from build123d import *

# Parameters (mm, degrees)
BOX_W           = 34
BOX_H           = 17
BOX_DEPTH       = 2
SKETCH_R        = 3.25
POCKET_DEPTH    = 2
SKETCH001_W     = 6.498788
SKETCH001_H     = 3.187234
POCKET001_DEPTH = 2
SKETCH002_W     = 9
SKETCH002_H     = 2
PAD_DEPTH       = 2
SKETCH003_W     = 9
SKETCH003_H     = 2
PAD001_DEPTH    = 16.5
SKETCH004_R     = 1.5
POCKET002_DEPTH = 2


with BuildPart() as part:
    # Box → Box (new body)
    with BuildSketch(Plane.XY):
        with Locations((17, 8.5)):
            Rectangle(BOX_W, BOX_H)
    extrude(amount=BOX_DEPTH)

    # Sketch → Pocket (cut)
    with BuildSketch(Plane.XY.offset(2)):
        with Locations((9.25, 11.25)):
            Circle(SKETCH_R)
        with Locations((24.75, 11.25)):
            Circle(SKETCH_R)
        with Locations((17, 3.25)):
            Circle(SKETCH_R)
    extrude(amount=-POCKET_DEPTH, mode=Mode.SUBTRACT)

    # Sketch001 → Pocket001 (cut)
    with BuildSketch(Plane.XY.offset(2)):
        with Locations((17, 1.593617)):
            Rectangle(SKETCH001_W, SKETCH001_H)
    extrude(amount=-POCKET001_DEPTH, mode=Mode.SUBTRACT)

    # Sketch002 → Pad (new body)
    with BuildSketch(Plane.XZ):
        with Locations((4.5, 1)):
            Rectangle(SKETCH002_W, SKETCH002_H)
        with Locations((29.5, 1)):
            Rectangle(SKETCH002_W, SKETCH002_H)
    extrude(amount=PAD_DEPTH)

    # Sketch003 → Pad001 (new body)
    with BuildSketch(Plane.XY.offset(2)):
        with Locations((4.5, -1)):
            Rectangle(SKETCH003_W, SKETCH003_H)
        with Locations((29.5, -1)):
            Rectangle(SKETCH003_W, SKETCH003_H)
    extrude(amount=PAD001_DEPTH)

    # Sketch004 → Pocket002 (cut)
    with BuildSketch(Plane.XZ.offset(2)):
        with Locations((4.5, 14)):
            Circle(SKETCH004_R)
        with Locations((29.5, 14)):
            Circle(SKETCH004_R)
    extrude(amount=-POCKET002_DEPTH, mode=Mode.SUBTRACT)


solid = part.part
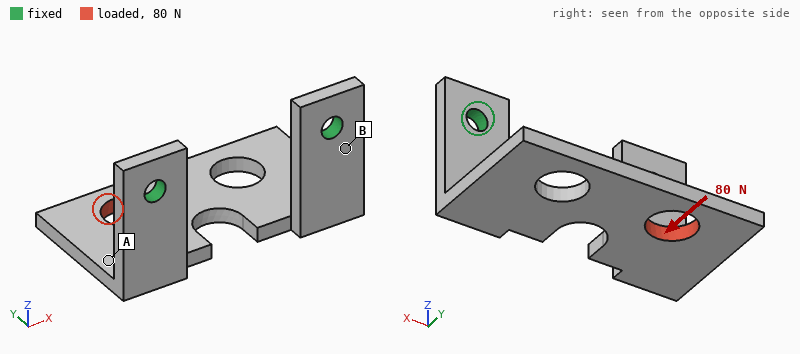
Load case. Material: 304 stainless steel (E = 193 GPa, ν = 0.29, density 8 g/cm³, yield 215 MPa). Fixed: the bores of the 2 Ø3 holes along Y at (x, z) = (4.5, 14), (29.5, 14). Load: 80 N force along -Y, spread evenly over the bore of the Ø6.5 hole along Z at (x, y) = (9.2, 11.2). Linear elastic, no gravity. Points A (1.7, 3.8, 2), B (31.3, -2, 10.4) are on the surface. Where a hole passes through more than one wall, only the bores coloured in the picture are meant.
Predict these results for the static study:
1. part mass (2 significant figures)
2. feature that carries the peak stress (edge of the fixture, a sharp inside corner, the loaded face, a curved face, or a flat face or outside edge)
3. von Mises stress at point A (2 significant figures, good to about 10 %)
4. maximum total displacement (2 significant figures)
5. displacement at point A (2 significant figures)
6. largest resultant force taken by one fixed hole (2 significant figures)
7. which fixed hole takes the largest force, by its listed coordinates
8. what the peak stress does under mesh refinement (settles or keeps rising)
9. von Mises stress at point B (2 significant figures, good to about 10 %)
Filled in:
13 g
edge of the fixture
13 MPa
62 µm
29 µm
60 N
(4.5, 14)
keeps rising
43 MPa
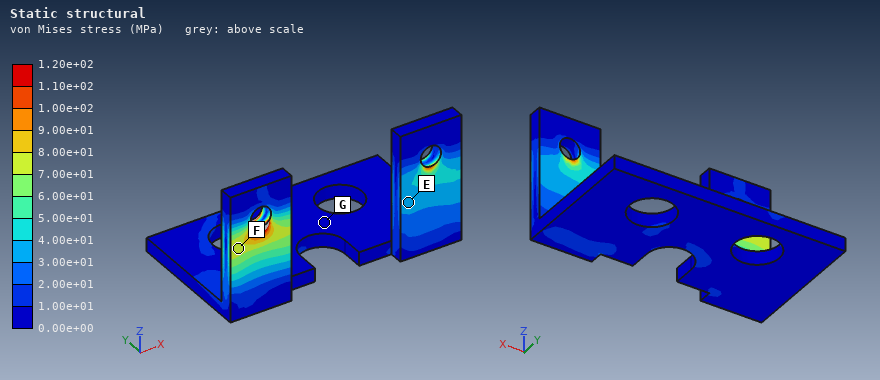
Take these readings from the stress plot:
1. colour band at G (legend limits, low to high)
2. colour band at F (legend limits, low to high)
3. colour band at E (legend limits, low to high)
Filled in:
0.00e+00 to 1.00e+01 MPa
7.00e+01 to 8.00e+01 MPa
3.00e+01 to 4.00e+01 MPa
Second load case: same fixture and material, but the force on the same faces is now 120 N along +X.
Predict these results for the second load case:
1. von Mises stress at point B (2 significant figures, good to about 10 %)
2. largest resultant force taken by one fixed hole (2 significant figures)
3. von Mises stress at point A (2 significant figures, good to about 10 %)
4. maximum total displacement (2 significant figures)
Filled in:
52 MPa
78 N
25 MPa
33 µm
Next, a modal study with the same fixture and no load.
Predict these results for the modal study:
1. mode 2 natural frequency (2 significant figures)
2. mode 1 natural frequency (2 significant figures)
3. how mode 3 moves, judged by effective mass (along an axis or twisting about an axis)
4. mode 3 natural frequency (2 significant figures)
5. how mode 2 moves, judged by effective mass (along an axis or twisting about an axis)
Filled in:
3700 Hz
1900 Hz
along Y
5600 Hz
along X
